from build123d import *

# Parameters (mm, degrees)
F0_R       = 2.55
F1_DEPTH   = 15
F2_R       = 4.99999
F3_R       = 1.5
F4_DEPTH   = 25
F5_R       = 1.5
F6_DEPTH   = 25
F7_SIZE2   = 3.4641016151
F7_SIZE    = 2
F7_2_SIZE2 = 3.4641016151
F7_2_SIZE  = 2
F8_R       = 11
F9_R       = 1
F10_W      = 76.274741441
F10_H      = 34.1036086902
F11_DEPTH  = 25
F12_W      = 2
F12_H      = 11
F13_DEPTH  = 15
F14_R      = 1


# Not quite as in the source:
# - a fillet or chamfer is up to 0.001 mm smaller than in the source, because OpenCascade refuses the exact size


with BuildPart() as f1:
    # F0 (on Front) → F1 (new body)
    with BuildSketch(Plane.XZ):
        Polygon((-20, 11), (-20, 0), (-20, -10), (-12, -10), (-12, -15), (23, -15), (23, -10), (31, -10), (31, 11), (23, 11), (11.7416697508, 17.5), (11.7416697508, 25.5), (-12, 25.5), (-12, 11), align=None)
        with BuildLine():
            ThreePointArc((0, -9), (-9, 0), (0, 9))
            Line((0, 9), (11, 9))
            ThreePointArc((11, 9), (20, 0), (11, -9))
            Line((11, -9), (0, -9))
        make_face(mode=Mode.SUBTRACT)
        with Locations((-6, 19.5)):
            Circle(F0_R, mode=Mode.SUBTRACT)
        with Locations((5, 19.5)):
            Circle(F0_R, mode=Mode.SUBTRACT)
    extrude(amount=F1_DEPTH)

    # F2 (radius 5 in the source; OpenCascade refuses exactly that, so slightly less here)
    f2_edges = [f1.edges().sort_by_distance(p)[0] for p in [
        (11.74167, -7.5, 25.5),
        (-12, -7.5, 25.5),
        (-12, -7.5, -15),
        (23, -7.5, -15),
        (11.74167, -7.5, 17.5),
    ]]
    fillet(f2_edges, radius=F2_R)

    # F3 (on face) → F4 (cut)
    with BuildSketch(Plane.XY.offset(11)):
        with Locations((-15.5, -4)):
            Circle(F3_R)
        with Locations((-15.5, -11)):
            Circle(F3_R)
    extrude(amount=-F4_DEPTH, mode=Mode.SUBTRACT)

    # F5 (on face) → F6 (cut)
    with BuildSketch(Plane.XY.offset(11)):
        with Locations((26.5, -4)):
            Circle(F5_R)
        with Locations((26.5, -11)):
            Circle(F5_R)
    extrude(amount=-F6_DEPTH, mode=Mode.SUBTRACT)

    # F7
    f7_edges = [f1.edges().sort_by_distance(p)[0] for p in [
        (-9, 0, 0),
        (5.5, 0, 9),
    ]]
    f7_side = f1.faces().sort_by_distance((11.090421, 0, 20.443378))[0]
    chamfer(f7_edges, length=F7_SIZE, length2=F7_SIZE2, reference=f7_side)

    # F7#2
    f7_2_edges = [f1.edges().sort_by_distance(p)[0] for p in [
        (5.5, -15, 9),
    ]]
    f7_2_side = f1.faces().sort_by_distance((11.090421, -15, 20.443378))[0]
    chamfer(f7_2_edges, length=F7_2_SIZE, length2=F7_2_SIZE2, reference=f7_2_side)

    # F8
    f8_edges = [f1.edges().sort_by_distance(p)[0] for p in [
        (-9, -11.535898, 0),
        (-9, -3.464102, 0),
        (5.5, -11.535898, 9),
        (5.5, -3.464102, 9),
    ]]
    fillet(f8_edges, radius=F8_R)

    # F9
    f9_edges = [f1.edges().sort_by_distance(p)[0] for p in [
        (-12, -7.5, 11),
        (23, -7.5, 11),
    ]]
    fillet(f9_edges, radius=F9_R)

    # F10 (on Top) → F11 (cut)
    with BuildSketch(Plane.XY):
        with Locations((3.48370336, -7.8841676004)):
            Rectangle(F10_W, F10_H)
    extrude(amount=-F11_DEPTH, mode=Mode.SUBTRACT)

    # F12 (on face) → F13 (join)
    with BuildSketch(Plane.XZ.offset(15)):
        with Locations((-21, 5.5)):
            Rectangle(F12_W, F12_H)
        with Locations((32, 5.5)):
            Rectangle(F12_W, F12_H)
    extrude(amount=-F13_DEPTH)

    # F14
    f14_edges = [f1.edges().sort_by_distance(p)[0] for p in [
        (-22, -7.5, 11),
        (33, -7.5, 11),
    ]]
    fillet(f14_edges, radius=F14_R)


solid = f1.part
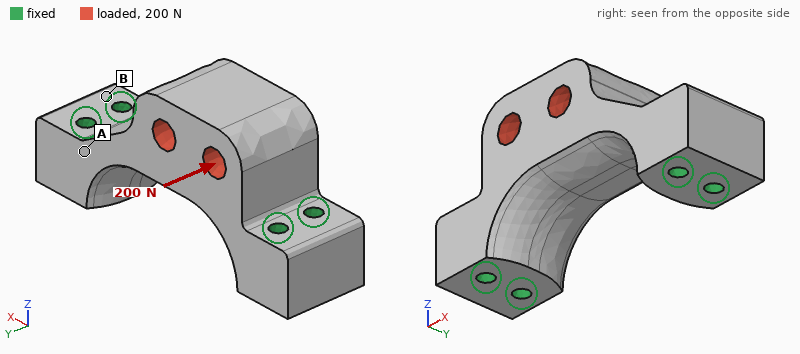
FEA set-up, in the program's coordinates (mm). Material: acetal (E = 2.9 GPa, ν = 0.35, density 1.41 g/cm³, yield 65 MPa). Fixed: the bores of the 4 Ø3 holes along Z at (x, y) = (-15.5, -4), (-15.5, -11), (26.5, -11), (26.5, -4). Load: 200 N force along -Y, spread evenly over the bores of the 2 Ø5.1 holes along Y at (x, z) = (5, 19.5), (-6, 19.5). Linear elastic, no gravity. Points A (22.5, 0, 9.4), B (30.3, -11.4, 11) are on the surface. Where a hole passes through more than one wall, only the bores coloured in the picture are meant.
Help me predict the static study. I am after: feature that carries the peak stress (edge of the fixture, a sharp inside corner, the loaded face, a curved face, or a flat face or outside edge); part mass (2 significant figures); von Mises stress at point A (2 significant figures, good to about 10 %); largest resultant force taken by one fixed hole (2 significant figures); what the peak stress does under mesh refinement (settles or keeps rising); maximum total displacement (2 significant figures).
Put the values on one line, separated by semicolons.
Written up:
edge of the fixture; 14 g; 3.7 MPa; 190 N; keeps rising; 92 µm
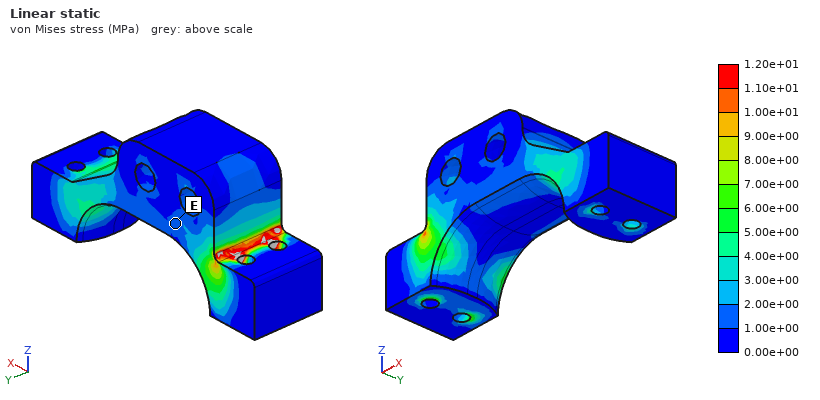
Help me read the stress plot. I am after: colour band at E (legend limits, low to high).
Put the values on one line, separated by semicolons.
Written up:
1.00e+00 to 2.00e+00 MPa
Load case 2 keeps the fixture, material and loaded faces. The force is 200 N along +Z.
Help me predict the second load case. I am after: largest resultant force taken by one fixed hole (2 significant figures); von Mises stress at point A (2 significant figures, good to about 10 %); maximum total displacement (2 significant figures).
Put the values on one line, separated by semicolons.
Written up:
78 N; 0.58 MPa; 15 µm
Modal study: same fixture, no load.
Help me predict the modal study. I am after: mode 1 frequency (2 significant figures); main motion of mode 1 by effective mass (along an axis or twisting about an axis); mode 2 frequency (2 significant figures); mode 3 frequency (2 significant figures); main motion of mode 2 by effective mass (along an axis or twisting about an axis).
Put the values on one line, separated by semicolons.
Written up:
3600 Hz; along Y; 6900 Hz; 8500 Hz; along Z
